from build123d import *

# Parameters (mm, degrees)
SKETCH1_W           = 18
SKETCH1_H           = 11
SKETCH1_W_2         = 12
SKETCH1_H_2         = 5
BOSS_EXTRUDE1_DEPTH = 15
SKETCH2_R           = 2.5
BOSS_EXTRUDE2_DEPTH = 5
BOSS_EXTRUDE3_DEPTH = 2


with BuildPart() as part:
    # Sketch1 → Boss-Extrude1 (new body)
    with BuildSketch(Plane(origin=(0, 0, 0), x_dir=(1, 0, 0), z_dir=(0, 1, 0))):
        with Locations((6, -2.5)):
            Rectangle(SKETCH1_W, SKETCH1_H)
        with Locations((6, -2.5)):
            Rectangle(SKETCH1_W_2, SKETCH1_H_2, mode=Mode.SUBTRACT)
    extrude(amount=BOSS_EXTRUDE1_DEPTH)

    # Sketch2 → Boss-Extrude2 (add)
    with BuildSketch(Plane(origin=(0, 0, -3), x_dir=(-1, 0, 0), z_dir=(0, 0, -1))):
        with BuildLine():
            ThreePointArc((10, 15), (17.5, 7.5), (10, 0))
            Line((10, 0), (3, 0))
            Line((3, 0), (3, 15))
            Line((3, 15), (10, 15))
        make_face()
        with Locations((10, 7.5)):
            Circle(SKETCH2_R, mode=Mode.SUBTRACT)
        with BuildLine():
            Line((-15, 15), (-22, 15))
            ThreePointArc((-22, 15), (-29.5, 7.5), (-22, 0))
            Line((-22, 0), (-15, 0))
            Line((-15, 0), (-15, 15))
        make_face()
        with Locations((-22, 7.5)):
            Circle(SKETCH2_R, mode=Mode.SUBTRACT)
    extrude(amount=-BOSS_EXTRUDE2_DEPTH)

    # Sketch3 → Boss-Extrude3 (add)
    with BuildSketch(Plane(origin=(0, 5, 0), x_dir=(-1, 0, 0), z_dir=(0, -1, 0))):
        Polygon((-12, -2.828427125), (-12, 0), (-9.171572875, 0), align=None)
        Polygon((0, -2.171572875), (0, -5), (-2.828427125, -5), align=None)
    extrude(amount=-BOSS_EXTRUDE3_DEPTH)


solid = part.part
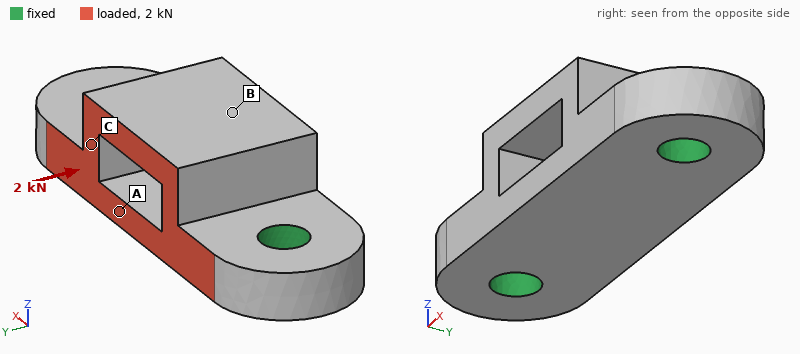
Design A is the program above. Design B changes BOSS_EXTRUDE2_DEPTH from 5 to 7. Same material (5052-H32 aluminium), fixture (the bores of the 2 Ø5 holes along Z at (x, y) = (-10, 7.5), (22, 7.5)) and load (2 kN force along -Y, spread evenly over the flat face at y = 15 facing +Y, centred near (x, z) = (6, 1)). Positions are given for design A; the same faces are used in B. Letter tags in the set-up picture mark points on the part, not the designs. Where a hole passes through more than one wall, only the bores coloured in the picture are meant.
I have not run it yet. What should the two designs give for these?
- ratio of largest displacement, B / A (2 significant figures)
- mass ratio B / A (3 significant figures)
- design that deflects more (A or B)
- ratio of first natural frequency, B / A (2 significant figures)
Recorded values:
0.51
1.18
A
1.4
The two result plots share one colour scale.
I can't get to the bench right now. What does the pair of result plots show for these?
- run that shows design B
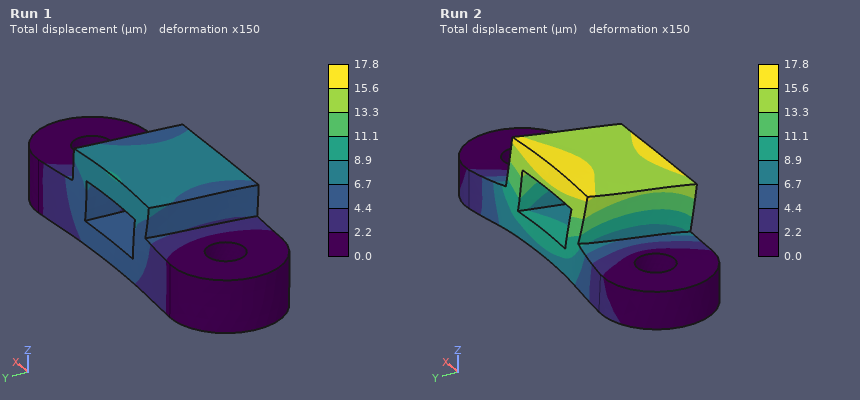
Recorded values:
Run 1
